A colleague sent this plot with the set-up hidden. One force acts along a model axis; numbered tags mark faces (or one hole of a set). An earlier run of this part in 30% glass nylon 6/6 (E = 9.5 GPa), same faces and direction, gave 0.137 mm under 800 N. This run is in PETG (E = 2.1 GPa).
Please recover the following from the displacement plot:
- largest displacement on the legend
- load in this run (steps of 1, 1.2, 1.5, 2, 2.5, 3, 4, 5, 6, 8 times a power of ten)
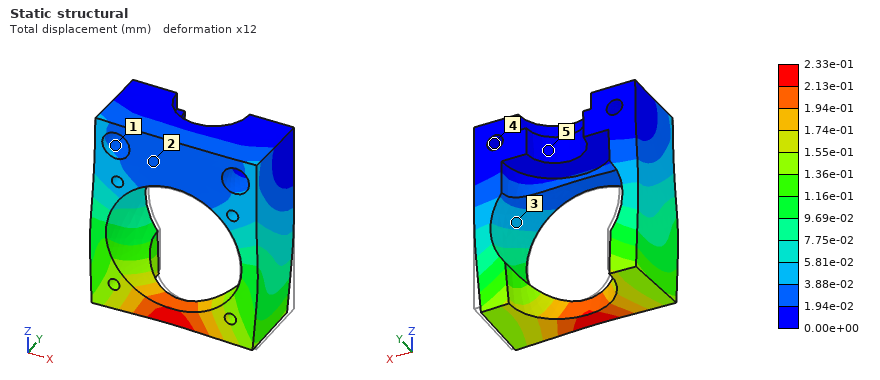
2.33e-01 mm
300 N
